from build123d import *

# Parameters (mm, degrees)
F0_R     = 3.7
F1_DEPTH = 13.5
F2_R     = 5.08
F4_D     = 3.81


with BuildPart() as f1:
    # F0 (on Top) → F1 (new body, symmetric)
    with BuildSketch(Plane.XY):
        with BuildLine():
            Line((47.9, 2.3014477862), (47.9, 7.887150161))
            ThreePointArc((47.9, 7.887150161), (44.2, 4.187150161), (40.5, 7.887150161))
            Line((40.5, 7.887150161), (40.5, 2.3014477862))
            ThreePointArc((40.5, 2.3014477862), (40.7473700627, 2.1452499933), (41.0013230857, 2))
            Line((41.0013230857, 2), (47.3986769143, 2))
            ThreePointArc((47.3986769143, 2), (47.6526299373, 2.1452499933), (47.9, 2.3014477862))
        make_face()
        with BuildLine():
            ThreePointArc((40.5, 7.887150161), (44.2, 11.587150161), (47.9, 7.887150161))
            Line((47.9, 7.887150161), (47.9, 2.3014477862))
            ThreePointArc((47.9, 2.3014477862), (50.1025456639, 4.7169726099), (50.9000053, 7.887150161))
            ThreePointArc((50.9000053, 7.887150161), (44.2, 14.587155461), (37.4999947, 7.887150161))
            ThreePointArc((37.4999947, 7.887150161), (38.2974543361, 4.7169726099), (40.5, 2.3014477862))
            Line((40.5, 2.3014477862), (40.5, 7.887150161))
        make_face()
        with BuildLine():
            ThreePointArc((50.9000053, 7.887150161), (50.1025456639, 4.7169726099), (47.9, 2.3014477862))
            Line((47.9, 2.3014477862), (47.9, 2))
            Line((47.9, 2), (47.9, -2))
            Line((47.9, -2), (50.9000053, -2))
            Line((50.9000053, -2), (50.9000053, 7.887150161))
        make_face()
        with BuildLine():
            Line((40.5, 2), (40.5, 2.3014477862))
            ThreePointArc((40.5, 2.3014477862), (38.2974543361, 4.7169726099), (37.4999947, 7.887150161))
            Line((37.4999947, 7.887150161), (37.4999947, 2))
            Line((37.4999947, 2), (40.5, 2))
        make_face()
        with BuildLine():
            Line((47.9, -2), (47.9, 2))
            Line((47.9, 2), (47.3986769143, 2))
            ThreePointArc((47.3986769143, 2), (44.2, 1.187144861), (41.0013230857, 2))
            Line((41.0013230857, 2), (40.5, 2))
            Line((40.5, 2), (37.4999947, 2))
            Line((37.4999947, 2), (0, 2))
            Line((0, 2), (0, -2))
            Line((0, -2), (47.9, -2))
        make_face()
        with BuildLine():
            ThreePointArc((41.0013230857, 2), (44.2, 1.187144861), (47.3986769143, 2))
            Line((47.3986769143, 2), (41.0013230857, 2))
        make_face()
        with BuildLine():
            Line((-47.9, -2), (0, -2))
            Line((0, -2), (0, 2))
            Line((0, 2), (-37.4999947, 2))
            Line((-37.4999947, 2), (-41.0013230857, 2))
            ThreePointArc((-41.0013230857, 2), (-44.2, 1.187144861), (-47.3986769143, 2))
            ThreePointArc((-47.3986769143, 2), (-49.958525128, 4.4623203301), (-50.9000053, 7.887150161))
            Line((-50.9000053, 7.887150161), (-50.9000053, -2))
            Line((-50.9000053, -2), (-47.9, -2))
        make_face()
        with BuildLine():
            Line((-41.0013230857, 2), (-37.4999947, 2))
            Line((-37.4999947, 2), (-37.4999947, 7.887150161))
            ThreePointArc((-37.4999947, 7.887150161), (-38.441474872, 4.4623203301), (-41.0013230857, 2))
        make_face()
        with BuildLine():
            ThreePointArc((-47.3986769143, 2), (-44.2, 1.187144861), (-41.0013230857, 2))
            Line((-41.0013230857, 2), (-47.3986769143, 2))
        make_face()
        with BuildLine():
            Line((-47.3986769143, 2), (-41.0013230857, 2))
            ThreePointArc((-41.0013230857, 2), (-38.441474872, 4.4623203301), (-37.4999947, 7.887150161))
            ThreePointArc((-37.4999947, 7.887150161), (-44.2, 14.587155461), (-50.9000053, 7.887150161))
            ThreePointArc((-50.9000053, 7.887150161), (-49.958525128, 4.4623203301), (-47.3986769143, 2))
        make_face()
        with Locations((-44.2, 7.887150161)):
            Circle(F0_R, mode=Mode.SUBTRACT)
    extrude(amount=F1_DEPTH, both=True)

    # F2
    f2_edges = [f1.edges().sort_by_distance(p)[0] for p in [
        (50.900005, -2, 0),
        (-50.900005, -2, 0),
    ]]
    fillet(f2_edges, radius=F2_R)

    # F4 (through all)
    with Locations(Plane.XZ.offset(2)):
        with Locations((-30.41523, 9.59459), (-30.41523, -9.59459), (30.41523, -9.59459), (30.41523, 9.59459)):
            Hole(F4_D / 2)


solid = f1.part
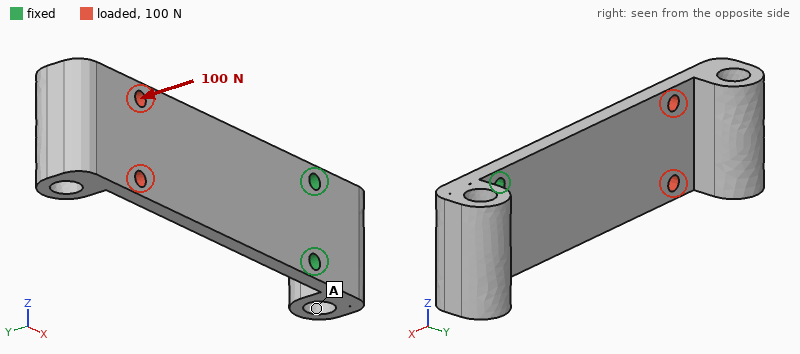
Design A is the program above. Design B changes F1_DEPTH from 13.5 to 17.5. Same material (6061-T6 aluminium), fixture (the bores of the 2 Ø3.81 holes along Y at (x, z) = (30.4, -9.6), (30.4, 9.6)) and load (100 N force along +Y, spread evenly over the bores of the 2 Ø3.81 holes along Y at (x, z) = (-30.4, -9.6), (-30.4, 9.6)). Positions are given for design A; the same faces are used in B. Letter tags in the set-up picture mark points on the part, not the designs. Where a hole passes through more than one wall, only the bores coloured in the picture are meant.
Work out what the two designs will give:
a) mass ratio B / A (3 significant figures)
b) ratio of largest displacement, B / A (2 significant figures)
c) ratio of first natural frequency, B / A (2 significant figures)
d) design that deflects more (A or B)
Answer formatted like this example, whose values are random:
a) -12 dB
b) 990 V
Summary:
a) 1.30
b) 0.77
c) 1.0
d) A
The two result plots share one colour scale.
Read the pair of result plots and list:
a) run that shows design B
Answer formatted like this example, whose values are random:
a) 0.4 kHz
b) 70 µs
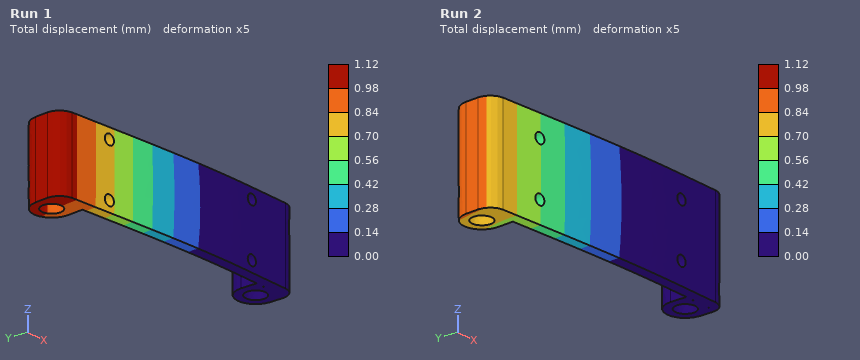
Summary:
a) Run 2
